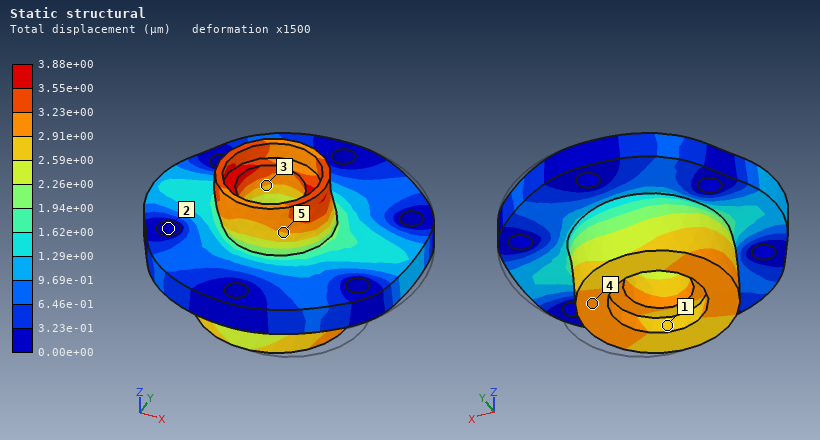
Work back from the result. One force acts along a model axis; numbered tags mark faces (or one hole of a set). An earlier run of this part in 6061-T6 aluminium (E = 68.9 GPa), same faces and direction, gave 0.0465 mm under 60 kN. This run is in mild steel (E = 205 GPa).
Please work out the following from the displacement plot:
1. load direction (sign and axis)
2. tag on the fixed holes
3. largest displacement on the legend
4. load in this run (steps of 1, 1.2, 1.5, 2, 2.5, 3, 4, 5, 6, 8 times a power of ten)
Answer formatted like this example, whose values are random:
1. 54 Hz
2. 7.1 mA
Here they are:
1. -X
2. 2
3. 3.88e+00 µm
4. 15 kN
